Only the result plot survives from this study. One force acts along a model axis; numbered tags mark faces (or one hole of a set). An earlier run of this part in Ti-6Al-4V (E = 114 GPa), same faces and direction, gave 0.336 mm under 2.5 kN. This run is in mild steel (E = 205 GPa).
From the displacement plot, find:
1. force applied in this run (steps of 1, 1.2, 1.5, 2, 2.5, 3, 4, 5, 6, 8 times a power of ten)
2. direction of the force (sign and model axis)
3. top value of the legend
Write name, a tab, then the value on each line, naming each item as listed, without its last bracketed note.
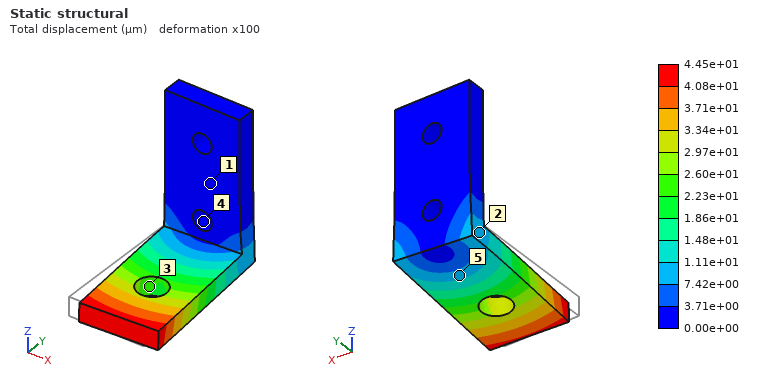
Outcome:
force applied in this run	600 N
direction of the force	+X
top value of the legend	4.45e+01 µm
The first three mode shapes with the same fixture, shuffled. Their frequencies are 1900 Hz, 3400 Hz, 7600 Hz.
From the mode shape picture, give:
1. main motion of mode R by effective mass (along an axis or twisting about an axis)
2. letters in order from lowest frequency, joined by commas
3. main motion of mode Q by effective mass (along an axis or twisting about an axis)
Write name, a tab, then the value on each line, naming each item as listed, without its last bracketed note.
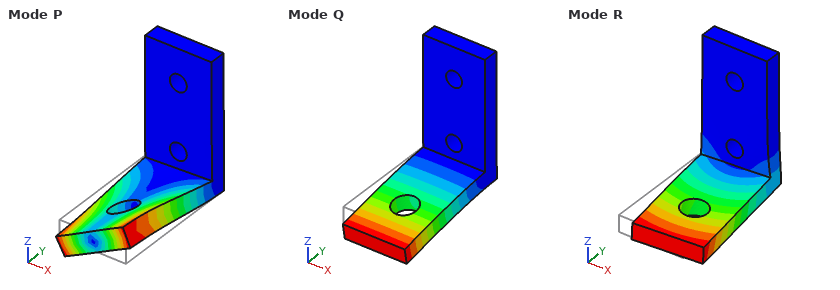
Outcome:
main motion of mode R by effective mass	along X
letters in order from lowest frequency, joined by commas	Q, R, P
main motion of mode Q by effective mass	along Z
